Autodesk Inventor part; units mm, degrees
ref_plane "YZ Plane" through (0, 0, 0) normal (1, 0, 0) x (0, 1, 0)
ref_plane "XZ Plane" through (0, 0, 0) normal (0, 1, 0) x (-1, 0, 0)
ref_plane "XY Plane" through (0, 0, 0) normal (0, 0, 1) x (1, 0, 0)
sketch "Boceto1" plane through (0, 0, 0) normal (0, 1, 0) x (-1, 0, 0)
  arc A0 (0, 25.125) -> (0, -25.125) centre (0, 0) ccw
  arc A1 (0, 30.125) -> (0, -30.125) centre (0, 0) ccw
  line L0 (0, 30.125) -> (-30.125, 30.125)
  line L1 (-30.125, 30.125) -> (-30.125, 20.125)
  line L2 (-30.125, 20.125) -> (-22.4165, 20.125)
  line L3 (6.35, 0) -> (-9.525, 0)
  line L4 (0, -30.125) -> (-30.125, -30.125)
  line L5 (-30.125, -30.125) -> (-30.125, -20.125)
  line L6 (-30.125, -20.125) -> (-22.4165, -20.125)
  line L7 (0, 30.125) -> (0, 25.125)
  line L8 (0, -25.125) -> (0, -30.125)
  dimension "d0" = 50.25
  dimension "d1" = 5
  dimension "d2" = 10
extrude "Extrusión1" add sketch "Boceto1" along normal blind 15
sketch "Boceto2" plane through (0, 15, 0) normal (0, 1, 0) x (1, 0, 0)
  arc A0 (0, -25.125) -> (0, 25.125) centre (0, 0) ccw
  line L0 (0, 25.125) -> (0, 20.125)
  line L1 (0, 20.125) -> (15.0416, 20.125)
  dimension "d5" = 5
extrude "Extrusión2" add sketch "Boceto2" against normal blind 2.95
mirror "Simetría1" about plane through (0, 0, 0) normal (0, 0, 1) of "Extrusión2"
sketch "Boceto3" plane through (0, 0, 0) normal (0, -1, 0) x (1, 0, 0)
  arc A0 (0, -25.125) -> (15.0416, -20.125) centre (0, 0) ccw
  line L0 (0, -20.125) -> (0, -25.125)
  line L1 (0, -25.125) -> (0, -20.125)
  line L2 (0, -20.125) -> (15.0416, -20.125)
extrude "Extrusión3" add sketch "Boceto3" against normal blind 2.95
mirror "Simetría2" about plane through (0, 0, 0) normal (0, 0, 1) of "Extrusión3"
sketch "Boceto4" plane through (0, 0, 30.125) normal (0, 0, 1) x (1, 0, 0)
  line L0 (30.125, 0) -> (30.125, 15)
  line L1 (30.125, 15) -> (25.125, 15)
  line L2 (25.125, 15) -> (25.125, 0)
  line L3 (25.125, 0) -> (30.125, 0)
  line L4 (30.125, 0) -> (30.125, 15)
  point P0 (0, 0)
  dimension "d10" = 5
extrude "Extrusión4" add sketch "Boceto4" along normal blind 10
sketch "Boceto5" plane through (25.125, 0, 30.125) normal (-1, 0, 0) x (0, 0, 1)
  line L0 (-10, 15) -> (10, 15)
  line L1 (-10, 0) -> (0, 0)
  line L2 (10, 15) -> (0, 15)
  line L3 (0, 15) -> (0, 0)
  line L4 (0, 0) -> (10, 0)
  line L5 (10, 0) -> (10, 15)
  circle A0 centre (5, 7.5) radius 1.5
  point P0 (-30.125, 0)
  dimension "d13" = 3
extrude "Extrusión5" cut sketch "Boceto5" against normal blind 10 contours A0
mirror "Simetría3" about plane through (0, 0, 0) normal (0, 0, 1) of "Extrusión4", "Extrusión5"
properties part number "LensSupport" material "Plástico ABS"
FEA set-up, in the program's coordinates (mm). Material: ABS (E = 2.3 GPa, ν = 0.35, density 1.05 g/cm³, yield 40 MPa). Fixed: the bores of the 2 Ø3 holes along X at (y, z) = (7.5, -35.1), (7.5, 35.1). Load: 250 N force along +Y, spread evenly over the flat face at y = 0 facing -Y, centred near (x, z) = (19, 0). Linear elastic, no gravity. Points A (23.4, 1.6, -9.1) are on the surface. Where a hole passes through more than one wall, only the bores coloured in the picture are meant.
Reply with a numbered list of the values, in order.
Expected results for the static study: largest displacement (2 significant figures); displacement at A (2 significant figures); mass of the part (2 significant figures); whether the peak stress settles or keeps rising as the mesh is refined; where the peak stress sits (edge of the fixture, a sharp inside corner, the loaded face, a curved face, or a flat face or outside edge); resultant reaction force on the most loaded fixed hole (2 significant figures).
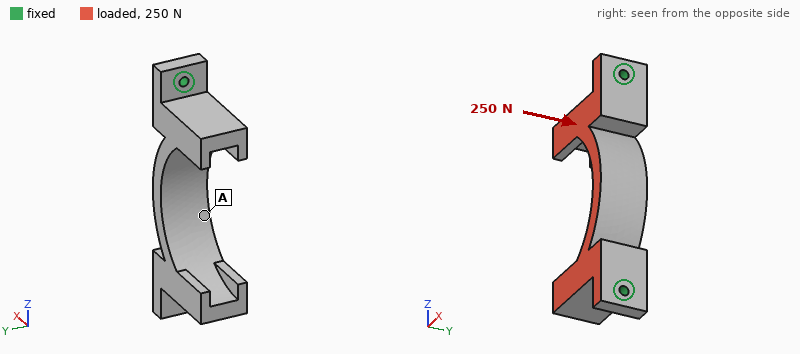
1. 0.62 mm
2. 0.25 mm
3. 14 g
4. keeps rising
5. edge of the fixture
6. 130 N
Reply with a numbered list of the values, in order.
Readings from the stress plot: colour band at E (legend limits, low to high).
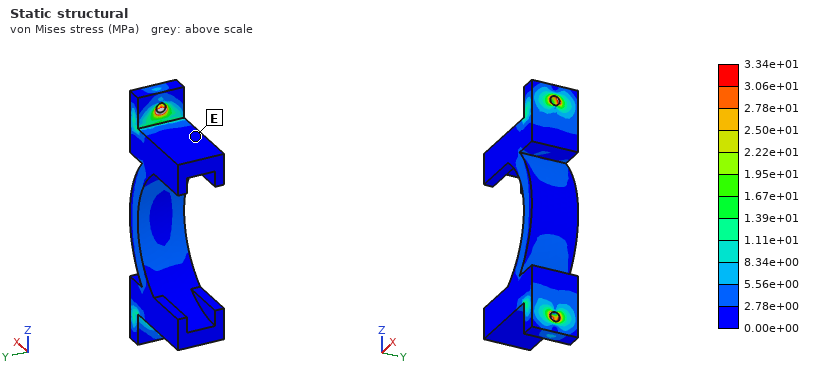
1. 0.00e+00 to 2.78e+00 MPa
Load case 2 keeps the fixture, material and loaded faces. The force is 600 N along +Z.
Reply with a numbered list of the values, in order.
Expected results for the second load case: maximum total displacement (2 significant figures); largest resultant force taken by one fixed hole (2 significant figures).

1. 0.71 mm
2. 310 N
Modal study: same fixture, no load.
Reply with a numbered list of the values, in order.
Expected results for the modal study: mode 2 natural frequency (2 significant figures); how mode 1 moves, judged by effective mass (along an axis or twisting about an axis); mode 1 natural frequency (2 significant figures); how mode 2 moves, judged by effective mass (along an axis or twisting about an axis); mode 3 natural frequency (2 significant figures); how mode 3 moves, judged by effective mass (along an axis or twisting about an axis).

1. 1200 Hz
2. along X
3. 980 Hz
4. along Y
5. 1400 Hz
6. twisting about X
